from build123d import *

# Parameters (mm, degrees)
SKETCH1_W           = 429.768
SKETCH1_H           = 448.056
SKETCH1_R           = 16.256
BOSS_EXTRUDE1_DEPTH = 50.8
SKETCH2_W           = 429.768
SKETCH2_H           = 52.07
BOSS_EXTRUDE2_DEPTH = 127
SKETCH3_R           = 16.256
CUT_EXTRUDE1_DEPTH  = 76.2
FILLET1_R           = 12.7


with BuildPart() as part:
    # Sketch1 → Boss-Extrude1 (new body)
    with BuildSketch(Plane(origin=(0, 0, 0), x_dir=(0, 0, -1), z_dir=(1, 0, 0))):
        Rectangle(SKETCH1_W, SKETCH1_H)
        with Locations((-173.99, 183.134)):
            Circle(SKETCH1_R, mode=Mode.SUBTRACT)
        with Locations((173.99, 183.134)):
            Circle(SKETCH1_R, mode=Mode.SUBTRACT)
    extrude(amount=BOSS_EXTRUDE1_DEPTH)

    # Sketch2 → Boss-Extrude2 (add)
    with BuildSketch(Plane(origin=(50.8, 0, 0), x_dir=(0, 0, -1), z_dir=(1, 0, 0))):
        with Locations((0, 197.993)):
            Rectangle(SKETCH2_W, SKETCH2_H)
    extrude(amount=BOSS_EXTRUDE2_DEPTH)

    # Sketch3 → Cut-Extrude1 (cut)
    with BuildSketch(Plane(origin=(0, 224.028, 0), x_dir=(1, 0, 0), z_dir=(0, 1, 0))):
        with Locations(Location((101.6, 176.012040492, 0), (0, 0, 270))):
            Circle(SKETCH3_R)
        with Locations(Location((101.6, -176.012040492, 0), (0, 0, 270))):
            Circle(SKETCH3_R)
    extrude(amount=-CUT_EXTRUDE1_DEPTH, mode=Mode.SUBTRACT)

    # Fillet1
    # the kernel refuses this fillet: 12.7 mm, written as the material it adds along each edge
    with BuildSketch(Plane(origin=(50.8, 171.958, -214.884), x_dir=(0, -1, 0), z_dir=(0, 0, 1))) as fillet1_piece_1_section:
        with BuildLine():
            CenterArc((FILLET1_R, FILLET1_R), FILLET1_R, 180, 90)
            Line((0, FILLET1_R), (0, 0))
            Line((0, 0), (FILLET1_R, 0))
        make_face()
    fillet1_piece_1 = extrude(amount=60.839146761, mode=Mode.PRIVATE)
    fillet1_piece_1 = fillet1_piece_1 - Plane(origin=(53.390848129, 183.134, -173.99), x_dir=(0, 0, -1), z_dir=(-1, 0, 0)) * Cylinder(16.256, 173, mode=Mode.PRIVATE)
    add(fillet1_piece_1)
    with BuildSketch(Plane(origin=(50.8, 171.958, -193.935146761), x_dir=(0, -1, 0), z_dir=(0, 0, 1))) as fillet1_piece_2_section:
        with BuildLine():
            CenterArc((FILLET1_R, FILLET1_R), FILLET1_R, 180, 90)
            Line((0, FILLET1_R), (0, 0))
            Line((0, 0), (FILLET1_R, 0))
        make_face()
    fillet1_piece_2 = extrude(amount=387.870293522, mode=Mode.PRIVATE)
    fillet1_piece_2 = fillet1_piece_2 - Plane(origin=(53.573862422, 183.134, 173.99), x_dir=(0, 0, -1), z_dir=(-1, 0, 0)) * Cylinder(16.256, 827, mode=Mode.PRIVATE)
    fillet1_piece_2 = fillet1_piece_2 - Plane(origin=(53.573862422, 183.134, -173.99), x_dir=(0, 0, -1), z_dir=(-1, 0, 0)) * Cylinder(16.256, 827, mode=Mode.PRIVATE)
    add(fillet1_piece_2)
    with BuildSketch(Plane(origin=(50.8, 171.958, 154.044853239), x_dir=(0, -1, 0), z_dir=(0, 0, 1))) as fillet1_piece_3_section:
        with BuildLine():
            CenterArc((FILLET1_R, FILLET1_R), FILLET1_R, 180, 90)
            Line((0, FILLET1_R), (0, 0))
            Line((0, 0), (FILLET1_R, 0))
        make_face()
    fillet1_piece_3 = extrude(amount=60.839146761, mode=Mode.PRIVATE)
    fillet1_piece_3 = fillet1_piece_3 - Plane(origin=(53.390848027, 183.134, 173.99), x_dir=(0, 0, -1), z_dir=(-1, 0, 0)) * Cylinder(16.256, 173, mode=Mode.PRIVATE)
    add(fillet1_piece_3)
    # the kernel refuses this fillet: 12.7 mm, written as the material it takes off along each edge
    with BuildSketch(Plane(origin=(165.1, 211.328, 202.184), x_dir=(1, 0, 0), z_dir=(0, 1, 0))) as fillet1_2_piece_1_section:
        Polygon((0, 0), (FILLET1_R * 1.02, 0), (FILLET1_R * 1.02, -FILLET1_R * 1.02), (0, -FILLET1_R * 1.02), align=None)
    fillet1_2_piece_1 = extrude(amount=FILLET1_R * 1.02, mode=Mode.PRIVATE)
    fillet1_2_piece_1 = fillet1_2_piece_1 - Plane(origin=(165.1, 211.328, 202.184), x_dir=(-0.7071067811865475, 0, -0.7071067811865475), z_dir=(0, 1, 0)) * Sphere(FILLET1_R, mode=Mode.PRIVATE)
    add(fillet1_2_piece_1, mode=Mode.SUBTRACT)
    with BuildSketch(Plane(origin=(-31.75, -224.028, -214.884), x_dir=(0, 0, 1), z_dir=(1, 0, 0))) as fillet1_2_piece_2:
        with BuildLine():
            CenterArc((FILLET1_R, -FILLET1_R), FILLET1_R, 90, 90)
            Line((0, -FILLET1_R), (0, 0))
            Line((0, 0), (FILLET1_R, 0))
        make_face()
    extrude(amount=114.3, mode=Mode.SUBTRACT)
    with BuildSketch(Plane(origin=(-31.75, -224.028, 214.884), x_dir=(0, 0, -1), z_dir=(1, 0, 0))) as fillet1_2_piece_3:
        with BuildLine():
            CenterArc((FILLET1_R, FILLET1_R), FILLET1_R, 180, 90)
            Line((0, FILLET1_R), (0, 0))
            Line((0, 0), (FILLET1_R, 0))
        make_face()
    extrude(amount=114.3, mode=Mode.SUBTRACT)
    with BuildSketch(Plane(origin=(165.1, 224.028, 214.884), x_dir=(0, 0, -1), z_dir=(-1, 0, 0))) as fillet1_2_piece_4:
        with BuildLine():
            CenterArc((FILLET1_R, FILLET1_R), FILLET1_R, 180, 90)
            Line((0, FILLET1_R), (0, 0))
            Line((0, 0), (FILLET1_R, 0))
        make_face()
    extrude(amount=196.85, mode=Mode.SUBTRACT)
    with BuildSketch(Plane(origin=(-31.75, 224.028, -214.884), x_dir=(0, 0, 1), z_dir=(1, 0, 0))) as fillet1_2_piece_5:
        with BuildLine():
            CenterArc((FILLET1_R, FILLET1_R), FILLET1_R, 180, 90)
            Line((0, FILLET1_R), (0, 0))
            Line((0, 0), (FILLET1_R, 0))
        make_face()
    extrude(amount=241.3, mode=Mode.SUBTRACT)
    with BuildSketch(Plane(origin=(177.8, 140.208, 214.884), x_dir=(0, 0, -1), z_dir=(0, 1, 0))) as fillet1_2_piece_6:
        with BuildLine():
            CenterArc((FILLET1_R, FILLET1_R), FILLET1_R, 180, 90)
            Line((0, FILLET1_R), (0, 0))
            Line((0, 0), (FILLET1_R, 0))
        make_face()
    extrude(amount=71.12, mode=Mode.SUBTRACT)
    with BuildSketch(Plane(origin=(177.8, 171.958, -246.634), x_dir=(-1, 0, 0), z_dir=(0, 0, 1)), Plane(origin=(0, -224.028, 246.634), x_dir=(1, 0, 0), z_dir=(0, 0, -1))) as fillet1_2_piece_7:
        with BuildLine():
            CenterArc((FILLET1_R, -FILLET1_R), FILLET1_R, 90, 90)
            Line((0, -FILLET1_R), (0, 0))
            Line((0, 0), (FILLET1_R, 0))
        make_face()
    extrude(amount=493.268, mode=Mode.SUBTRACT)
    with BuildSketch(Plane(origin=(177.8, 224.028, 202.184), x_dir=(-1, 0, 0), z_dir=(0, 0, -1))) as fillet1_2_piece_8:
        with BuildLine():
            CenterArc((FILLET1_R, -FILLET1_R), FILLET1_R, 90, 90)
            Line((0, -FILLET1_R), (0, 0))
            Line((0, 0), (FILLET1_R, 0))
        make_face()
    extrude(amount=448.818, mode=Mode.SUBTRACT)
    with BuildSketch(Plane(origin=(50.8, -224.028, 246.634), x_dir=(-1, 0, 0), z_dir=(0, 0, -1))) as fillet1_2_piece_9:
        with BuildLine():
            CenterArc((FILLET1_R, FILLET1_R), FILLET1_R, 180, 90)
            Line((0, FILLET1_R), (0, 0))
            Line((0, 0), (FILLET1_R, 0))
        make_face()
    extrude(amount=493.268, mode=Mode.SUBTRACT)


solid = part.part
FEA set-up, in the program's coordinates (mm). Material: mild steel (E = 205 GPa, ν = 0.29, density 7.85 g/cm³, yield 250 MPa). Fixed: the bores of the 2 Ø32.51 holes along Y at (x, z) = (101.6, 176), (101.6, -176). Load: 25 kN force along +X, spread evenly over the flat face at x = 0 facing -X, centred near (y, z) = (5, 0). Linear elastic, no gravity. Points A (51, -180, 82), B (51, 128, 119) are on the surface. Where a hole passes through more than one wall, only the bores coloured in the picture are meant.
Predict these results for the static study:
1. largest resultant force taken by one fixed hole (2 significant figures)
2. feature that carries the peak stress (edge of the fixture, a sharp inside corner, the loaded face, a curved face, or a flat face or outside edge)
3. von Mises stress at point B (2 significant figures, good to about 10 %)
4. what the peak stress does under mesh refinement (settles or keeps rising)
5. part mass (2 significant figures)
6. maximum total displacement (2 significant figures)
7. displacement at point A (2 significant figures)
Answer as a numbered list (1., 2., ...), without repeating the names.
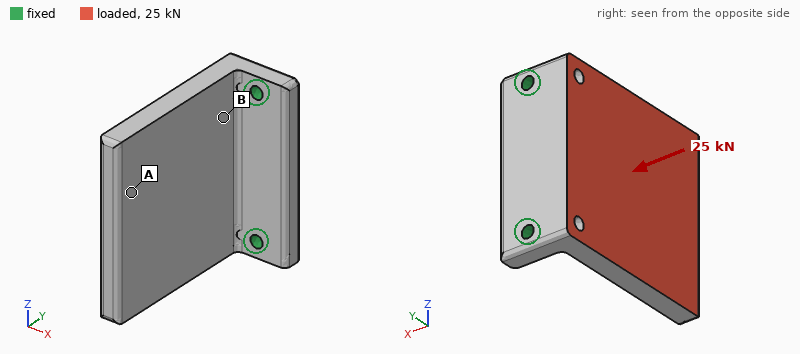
1. 13 kN
2. a sharp inside corner
3. 17 MPa
4. keeps rising
5. 97 kg
6. 0.40 mm
7. 0.34 mm
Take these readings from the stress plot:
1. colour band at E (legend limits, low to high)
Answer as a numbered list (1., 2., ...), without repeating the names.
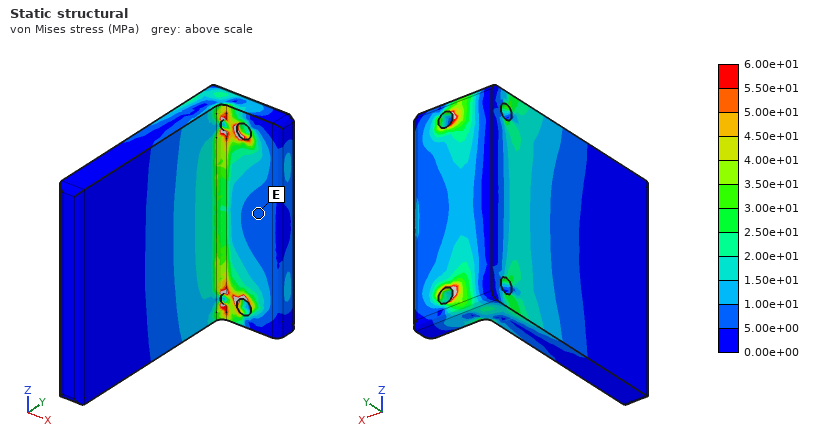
1. 5.00e+00 to 1.00e+01 MPa
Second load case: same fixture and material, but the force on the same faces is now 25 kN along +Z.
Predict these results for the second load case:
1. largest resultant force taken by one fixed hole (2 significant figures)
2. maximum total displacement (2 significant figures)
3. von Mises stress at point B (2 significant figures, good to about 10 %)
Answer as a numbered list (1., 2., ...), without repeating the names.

1. 20 kN
2. 21 µm
3. 3.7 MPa
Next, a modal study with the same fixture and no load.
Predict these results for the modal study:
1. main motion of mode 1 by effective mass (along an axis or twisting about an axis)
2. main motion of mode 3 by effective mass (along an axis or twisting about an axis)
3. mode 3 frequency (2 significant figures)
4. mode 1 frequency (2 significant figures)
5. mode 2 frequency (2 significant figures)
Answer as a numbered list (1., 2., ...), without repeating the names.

1. along X
2. along Z
3. 740 Hz
4. 180 Hz
5. 490 Hz
